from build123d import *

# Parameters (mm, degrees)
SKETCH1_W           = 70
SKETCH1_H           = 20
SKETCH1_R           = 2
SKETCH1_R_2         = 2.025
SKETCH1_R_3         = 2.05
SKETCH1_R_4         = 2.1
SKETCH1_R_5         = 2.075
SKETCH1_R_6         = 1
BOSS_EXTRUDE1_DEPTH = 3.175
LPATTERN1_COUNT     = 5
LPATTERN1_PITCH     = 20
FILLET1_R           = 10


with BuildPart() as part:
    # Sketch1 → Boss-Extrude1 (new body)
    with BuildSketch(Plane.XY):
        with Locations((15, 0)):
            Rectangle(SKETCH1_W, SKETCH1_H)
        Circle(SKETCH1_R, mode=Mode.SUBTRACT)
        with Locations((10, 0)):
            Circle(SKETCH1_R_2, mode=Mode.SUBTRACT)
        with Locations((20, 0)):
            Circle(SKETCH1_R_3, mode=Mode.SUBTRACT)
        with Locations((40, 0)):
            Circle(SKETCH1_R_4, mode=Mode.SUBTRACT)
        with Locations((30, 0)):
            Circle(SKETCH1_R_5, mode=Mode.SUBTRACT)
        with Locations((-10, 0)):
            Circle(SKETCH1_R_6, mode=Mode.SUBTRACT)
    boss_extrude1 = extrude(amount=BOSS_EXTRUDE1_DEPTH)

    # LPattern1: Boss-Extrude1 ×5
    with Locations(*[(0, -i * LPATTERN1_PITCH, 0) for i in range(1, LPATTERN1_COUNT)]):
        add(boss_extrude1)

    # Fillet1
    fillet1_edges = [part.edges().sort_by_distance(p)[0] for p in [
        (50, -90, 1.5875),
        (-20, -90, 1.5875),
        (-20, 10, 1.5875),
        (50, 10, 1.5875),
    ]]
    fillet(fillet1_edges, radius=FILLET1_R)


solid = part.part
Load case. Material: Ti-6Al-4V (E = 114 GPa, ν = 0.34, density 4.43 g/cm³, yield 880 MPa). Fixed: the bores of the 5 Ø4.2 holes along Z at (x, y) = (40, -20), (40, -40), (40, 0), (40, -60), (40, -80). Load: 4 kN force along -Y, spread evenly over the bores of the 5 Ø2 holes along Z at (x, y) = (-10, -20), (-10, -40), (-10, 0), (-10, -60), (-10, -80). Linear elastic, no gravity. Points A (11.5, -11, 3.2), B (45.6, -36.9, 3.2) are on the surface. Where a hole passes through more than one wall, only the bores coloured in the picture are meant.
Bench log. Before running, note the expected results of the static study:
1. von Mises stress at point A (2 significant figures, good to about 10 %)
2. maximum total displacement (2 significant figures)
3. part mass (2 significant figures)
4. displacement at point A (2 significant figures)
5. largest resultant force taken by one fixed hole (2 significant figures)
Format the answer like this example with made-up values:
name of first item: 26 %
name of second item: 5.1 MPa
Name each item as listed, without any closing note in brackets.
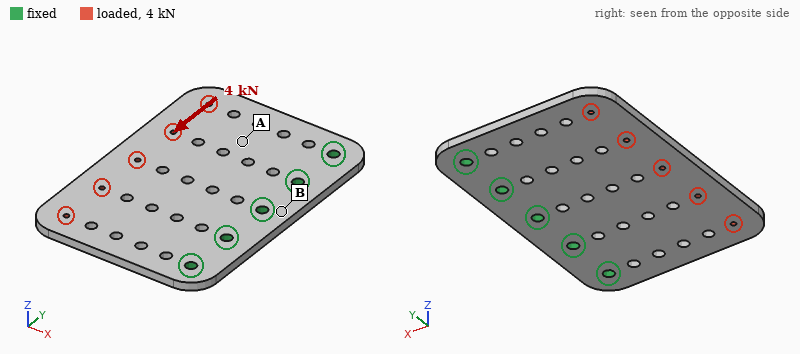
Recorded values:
von Mises stress at point A: 27 MPa
maximum total displacement: 34 µm
part mass: 92 g
displacement at point A: 16 µm
largest resultant force taken by one fixed hole: 2.3 kN
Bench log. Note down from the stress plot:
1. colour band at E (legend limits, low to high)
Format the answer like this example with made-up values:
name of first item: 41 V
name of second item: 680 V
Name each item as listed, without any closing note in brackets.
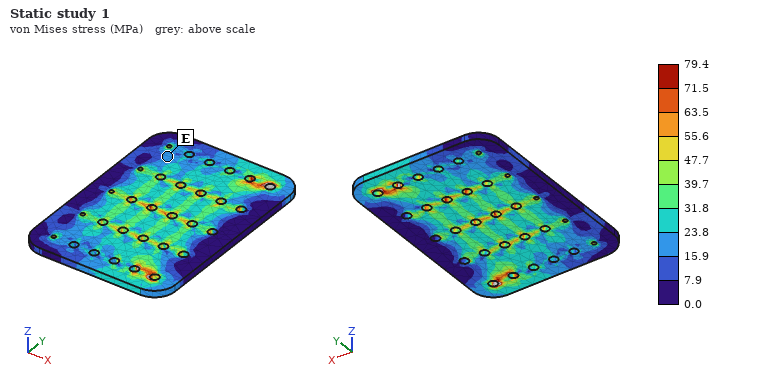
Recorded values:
colour band at E: 15.9 to 23.8 MPa
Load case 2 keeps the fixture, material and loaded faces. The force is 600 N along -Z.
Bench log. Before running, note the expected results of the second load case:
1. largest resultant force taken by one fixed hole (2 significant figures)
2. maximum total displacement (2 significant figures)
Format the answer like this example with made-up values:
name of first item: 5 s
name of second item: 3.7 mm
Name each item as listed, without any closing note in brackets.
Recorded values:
largest resultant force taken by one fixed hole: 160 N
maximum total displacement: 1.1 mm
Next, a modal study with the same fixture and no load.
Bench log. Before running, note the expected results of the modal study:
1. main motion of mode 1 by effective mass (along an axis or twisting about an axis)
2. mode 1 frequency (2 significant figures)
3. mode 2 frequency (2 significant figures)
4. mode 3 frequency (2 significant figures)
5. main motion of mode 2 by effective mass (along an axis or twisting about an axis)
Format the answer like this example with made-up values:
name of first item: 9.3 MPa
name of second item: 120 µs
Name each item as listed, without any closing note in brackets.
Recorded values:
main motion of mode 1 by effective mass: along Z
mode 1 frequency: 730 Hz
mode 2 frequency: 1300 Hz
mode 3 frequency: 2700 Hz
main motion of mode 2 by effective mass: twisting about X
